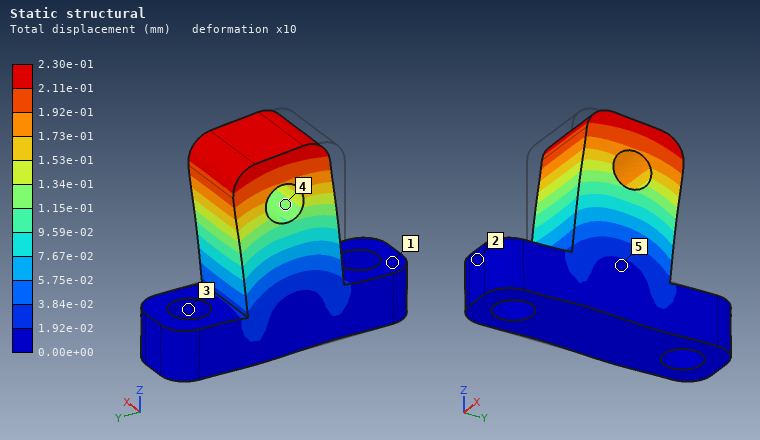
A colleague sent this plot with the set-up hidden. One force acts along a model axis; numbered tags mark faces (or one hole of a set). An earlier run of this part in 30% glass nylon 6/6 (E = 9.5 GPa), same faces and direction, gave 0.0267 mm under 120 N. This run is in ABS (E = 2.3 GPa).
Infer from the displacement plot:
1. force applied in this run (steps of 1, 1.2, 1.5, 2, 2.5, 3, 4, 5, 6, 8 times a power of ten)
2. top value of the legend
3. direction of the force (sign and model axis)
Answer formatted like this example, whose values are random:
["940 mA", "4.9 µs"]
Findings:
["250 N", "2.30e-01 mm", "+Y"]
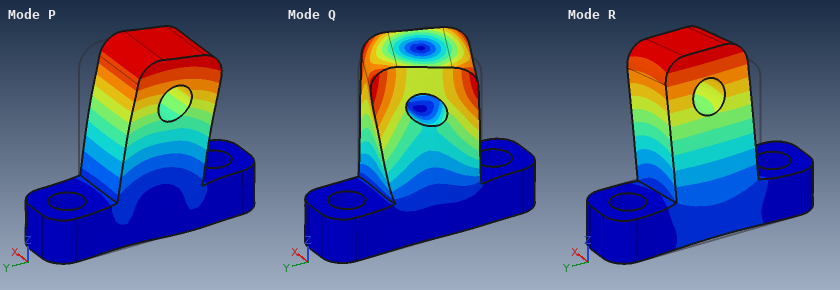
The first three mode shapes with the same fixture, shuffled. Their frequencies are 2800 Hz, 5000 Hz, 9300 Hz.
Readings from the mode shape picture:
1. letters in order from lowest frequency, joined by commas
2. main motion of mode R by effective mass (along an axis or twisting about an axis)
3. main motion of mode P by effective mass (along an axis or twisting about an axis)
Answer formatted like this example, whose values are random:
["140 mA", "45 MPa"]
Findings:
["R, P, Q", "along X", "along Y"]
